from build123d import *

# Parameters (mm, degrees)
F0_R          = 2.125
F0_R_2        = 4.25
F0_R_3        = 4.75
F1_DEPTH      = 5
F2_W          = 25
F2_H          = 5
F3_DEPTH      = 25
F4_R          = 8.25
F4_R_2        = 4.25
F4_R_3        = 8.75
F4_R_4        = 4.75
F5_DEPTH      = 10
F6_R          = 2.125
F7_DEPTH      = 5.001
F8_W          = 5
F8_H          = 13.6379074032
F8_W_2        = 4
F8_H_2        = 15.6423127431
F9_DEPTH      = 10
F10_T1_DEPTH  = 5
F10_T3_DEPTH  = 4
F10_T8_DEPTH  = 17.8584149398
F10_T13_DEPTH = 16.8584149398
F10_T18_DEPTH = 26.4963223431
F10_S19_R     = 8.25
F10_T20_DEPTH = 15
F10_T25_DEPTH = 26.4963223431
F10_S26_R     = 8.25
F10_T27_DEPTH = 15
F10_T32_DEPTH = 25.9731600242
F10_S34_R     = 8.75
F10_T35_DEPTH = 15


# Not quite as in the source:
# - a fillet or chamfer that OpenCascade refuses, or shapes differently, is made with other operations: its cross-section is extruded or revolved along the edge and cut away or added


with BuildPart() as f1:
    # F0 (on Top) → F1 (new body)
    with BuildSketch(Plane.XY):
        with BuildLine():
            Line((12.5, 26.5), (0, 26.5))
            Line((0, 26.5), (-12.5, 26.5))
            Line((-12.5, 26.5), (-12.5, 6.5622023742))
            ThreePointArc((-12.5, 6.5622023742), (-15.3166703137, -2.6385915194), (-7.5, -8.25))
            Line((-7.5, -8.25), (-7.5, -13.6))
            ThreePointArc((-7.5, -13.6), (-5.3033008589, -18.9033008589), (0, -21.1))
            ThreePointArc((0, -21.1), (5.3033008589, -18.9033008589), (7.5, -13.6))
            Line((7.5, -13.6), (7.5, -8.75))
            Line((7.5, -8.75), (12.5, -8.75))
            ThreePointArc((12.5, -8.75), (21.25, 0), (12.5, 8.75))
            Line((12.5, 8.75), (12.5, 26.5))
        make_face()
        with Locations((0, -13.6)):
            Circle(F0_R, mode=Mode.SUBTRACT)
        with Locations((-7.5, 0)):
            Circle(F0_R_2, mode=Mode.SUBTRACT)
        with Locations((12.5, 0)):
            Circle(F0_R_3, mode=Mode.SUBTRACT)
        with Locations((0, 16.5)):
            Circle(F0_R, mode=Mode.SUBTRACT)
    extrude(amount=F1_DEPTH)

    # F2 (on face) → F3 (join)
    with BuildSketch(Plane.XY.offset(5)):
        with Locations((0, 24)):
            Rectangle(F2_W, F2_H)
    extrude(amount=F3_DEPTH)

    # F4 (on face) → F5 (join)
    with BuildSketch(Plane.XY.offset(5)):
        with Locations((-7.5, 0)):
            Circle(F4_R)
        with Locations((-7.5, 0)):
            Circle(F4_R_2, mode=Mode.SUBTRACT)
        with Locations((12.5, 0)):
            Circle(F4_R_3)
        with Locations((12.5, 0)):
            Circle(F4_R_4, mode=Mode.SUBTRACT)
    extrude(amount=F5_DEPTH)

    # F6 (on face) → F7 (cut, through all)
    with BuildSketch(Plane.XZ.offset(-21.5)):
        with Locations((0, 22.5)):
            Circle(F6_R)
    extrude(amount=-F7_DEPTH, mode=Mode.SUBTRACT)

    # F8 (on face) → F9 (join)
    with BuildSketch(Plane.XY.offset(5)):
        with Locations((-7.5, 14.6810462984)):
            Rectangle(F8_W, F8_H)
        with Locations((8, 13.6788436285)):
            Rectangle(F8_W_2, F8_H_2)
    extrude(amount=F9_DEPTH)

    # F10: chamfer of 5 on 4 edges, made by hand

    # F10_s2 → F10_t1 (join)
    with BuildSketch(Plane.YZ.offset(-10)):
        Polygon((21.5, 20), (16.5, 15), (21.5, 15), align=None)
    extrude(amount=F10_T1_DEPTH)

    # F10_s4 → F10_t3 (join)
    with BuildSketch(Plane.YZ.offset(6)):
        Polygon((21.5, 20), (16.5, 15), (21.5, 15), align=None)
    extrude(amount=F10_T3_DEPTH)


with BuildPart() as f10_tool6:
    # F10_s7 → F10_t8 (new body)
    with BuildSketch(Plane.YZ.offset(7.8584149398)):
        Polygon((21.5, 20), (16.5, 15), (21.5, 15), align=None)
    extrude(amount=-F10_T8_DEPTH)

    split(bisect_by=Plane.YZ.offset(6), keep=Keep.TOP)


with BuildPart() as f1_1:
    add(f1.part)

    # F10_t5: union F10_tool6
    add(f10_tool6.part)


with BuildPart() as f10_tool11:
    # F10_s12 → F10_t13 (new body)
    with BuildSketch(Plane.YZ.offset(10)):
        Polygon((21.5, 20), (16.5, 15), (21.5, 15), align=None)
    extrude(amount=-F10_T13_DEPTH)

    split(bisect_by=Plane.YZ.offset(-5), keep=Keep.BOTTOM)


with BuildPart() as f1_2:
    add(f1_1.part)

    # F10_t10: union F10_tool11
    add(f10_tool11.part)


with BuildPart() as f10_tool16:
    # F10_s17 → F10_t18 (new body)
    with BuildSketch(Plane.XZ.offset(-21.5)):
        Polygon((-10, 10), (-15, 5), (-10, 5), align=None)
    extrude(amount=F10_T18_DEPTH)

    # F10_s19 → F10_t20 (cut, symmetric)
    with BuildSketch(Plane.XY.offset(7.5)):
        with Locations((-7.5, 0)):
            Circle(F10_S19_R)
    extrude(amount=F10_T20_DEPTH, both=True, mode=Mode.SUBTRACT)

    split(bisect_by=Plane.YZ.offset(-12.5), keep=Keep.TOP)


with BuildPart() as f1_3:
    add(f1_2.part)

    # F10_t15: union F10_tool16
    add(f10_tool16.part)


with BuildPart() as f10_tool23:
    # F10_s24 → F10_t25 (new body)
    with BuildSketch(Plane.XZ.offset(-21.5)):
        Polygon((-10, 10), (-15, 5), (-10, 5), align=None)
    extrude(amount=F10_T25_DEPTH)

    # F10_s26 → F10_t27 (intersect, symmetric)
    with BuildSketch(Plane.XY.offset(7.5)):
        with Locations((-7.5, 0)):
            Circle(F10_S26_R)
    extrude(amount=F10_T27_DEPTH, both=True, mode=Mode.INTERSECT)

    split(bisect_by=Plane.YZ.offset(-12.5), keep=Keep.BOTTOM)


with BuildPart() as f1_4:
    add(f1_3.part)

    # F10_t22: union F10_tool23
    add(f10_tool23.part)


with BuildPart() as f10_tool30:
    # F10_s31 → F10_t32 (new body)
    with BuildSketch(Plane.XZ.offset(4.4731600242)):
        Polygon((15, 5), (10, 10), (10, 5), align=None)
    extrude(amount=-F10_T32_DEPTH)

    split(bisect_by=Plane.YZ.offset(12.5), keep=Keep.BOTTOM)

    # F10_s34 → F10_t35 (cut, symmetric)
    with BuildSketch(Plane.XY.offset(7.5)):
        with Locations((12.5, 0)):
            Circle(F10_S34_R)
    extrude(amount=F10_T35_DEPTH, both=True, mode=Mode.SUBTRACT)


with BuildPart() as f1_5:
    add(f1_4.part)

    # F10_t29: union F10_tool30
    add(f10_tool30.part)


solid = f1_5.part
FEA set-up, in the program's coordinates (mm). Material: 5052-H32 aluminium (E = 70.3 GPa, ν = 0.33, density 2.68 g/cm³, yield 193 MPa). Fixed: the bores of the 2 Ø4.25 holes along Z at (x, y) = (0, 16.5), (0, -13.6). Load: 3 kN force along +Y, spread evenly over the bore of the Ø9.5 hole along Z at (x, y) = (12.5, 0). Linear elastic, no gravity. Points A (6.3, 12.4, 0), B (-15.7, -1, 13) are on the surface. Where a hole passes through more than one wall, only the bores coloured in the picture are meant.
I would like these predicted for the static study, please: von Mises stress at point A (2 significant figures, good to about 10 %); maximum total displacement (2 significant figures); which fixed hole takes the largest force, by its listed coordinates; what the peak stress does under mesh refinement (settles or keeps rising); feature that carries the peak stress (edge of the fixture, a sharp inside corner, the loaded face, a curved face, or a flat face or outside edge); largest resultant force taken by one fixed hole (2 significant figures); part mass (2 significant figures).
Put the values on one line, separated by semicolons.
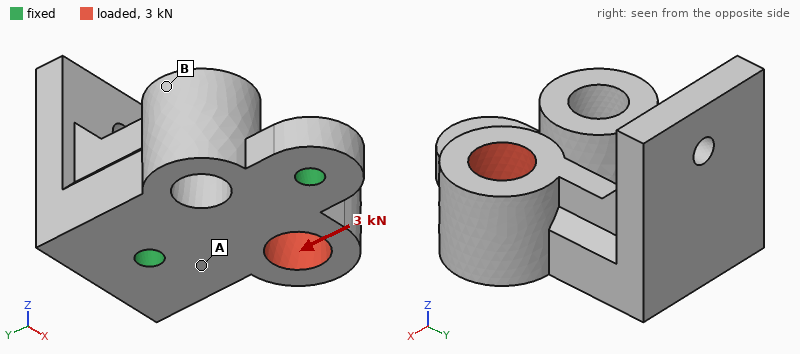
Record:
25 MPa; 31 µm; (0, 16.5); keeps rising; a sharp inside corner; 2.1 kN; 35 g
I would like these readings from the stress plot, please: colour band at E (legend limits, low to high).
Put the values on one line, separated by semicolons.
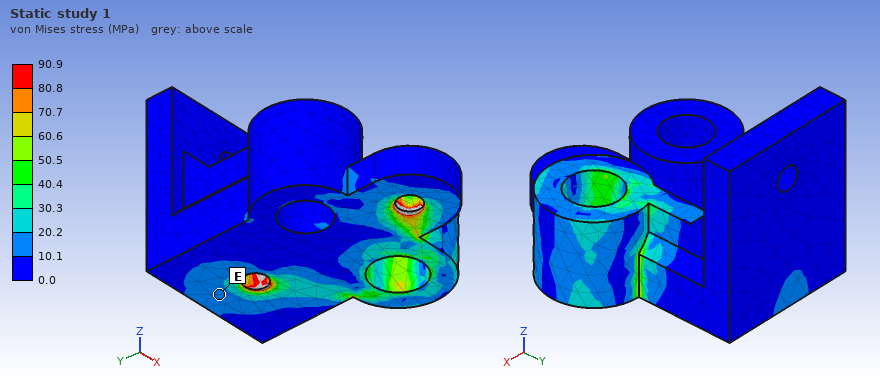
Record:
10.1 to 20.2 MPa
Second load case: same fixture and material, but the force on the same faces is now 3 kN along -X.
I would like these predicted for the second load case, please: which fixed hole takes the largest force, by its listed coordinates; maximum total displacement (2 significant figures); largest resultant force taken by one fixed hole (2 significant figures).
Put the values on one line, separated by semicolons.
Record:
(0, -13.6); 0.11 mm; 1.7 kN
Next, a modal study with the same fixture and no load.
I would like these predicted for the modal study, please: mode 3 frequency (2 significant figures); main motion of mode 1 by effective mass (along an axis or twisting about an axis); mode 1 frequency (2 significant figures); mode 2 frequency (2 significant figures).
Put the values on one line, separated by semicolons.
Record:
11 kHz; along X; 5600 Hz; 9300 Hz
